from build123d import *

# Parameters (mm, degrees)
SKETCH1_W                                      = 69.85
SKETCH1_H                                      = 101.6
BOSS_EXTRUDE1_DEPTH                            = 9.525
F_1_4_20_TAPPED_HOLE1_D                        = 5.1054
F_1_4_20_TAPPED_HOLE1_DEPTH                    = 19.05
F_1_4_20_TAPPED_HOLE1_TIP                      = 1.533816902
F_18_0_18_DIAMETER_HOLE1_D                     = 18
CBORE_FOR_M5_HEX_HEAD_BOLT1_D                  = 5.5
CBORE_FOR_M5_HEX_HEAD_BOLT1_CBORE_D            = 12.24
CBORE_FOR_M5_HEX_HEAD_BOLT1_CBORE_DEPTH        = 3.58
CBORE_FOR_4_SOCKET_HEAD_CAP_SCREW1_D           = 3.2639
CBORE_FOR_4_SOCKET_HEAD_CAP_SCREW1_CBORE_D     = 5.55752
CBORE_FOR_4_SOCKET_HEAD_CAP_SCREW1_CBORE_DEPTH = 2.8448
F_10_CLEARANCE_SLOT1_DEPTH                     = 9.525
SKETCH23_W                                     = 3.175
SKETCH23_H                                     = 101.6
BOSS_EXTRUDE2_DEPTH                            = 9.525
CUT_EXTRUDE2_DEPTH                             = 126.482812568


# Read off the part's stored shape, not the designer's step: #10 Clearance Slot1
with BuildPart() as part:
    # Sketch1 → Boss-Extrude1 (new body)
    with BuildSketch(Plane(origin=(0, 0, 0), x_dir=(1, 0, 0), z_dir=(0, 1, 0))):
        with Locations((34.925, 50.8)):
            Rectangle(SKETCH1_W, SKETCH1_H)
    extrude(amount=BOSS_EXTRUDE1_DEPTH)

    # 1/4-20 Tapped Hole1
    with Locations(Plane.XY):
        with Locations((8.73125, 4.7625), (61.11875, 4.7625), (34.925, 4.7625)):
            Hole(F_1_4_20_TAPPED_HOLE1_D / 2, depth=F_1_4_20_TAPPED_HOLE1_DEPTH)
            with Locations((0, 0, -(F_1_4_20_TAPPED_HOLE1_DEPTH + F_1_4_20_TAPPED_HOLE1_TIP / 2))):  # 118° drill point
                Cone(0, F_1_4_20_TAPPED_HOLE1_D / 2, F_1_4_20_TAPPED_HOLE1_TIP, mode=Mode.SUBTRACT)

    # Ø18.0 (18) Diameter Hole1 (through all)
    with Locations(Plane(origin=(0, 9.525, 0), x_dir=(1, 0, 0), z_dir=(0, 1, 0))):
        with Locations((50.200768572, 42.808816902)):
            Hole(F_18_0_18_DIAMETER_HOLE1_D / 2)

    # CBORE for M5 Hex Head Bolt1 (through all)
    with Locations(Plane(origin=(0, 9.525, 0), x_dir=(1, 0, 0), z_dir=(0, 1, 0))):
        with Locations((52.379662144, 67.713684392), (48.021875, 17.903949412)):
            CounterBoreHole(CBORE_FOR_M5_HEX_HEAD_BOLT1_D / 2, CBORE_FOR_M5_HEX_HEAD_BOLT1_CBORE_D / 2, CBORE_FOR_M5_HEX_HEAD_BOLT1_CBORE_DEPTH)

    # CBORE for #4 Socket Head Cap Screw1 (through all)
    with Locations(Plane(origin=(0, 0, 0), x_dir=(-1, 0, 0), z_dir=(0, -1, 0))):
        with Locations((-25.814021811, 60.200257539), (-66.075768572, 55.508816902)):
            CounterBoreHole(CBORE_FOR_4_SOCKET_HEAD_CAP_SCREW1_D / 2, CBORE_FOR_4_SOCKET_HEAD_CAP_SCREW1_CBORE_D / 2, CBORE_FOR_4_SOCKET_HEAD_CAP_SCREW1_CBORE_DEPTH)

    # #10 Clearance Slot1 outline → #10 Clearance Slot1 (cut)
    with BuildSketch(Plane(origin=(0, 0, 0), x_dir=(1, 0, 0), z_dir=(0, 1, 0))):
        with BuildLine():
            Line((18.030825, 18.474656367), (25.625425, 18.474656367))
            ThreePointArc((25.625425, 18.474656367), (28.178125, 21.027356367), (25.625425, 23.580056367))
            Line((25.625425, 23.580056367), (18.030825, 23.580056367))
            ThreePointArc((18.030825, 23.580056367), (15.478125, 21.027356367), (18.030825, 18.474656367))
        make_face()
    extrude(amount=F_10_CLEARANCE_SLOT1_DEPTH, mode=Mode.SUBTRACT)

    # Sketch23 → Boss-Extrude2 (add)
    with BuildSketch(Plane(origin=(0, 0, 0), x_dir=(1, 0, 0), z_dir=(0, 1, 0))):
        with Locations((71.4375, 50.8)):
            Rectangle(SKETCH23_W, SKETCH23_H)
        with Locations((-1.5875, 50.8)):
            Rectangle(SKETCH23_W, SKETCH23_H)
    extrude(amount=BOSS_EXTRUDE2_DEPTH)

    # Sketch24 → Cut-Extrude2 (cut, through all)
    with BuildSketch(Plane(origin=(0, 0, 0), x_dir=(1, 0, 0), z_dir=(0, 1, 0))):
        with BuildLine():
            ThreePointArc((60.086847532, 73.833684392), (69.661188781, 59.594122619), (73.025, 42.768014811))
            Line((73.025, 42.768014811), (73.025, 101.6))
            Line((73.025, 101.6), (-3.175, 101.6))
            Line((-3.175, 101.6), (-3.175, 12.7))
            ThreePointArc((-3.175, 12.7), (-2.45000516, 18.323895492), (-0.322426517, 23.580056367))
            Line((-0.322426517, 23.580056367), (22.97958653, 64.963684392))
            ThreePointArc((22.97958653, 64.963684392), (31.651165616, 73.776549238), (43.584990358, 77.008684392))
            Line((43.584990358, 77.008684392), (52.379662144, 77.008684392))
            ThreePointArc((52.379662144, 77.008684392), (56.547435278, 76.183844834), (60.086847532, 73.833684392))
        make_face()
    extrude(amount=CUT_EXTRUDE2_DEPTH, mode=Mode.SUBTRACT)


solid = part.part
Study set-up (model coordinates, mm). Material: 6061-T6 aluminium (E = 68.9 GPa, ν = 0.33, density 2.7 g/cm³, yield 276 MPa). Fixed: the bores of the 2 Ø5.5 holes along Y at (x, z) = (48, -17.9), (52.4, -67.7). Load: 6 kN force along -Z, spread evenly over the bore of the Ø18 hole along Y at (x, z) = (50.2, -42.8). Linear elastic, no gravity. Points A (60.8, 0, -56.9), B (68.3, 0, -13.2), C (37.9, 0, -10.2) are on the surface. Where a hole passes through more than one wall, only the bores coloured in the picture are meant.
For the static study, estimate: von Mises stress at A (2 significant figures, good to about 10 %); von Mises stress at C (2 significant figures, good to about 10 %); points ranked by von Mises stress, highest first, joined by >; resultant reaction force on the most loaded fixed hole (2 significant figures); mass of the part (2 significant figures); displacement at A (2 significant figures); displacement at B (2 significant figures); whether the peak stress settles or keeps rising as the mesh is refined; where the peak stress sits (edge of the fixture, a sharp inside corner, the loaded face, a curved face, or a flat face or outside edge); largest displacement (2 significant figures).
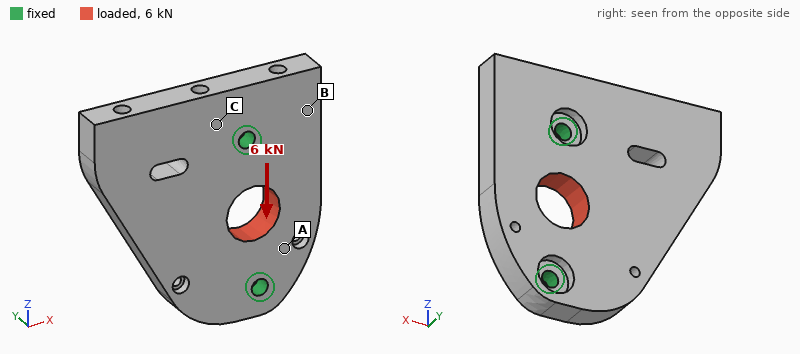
15 MPa
8.1 MPa
A > C > B
3.1 kN
110 g
4.0 µm
4.3 µm
keeps rising
edge of the fixture
6.9 µm
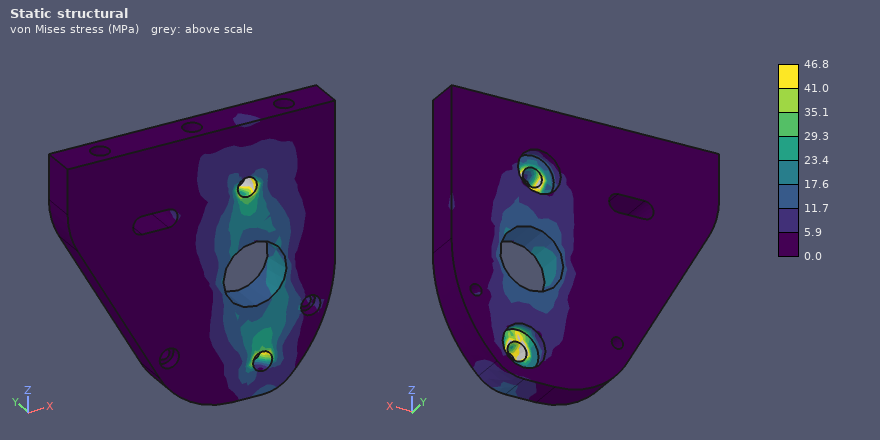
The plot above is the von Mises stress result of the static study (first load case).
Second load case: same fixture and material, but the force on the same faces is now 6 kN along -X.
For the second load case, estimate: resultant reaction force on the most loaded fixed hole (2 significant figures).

3.0 kN
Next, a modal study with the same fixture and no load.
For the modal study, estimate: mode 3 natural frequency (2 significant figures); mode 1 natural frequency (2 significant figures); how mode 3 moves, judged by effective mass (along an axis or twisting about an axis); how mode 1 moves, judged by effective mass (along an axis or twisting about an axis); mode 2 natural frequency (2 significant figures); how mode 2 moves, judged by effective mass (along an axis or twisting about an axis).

7700 Hz
2400 Hz
along Y
along Y
5900 Hz
twisting about X
